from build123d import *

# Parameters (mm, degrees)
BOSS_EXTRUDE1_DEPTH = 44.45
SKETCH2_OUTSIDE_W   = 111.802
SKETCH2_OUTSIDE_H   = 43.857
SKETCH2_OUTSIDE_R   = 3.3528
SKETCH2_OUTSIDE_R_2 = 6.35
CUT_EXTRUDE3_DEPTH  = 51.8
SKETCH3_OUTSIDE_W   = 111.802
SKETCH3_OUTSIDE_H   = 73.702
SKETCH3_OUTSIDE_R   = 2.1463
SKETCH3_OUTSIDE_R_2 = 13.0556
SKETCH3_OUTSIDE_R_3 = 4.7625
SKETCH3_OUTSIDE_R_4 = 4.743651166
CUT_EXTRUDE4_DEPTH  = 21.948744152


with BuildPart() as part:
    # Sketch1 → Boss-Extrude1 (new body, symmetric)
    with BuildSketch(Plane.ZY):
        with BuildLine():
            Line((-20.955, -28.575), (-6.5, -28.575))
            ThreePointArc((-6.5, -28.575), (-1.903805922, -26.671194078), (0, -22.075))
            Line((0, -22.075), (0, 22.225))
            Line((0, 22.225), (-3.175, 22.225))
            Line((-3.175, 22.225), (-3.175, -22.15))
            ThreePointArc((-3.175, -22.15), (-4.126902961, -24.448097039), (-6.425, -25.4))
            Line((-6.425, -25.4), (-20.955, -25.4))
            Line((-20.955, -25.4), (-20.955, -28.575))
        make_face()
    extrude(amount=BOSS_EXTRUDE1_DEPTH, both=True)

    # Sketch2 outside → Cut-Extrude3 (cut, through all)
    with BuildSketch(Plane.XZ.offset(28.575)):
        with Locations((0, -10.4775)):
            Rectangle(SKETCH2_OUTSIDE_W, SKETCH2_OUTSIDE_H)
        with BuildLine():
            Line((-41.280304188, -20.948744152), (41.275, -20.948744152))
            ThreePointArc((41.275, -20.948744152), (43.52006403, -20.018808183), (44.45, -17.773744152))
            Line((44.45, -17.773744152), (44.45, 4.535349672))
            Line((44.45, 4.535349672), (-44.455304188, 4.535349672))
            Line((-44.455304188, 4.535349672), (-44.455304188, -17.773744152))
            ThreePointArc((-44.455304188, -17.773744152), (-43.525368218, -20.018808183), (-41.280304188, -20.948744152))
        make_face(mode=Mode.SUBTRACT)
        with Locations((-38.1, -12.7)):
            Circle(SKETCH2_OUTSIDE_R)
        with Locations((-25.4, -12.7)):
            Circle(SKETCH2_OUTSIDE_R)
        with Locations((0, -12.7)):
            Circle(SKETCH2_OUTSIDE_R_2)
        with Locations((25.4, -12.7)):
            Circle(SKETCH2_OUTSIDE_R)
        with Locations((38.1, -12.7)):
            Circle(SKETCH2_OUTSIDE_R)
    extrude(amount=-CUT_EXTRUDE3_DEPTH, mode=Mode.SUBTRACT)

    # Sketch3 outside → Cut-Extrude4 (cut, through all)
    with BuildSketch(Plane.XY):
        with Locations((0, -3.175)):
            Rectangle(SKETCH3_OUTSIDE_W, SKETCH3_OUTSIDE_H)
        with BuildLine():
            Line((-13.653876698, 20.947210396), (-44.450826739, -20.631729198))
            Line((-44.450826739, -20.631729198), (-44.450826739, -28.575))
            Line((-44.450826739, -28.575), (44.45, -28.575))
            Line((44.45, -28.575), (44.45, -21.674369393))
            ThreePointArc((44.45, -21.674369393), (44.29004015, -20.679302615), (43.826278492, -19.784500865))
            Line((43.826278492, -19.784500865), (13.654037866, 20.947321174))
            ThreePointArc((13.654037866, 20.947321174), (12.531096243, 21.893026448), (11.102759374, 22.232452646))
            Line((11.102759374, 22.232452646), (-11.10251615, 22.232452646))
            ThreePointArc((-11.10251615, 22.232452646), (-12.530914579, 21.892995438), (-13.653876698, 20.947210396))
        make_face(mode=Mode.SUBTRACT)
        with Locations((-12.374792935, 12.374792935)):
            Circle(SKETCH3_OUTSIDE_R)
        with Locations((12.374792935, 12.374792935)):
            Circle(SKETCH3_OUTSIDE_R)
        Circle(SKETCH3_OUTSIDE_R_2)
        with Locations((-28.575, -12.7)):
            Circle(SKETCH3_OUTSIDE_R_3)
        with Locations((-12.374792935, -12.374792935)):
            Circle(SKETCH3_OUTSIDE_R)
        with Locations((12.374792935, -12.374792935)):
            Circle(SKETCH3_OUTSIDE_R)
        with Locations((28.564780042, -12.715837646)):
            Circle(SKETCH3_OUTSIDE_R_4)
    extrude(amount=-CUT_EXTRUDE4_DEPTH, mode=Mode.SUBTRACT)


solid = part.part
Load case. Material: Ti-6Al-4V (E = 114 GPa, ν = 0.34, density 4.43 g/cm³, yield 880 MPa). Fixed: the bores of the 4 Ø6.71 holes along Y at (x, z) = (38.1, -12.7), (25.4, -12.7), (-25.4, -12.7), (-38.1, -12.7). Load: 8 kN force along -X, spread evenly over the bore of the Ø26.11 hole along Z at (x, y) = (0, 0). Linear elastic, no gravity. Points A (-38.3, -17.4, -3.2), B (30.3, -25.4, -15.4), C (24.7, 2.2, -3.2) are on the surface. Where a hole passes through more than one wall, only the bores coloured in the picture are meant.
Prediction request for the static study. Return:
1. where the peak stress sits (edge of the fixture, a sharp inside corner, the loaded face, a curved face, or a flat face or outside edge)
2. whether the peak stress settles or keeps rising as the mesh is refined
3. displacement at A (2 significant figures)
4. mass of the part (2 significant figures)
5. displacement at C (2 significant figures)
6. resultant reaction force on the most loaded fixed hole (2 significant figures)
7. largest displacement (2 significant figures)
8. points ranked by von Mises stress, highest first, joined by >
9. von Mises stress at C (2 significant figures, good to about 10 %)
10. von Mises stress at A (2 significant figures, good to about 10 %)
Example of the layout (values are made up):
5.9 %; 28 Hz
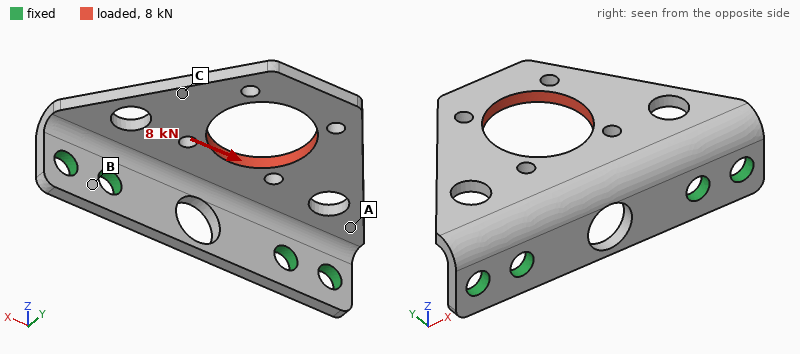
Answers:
edge of the fixture; keeps rising; 0.14 mm; 50 g; 0.21 mm; 3.0 kN; 0.24 mm; A > C > B; 98 MPa; 150 MPa
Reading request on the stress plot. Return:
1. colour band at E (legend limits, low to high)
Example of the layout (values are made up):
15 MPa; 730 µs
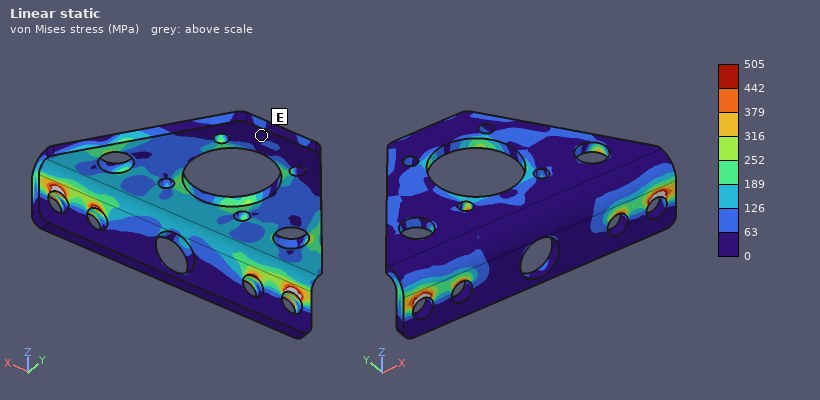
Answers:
0 to 63 MPa
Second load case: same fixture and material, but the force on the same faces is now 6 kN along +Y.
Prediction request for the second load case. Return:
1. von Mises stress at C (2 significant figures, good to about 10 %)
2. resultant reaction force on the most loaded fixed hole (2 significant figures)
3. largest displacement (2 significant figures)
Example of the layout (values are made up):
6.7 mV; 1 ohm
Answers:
60 MPa; 2.1 kN; 0.59 mm
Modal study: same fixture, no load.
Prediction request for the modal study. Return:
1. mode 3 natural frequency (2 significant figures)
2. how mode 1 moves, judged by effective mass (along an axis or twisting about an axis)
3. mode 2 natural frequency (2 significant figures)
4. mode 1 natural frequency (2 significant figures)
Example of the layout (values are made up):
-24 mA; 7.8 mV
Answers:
4800 Hz; along Z; 2900 Hz; 1200 Hz
